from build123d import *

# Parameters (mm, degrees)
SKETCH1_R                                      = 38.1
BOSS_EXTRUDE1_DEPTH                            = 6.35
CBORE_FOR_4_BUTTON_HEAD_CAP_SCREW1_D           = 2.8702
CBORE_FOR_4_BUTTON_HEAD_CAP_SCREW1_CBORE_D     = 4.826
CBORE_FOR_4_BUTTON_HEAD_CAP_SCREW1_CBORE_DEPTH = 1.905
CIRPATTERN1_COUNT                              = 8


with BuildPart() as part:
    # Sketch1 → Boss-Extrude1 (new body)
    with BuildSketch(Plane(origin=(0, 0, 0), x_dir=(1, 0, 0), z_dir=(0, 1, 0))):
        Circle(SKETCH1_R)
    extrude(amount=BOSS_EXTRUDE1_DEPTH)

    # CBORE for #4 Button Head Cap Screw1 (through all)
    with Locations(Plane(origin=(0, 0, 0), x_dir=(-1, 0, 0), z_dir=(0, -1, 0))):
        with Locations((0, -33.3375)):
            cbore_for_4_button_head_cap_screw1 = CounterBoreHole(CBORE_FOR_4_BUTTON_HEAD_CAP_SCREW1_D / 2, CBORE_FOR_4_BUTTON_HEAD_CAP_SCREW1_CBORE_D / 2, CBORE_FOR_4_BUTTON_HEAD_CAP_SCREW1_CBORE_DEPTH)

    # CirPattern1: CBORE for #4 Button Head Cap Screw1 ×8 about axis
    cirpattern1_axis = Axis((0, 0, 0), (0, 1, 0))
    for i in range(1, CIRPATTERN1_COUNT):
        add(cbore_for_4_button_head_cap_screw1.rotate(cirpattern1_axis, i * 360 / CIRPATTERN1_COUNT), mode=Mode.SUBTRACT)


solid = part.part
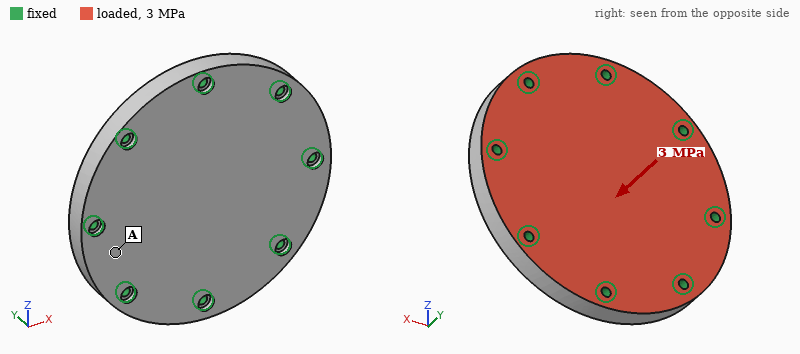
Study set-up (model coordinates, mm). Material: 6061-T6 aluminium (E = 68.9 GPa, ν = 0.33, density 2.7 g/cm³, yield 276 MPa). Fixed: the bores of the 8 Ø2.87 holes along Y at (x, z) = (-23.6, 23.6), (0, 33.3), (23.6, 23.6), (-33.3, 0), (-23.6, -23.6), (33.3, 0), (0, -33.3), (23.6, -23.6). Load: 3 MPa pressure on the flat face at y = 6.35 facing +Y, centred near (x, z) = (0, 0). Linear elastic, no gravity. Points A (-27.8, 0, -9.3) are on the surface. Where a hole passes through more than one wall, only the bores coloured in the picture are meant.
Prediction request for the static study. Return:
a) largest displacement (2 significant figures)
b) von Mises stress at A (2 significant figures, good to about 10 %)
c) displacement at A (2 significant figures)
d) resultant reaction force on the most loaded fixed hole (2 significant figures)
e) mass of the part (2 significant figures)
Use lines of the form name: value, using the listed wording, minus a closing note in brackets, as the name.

largest displacement: 70 µm
von Mises stress at A: 36 MPa
displacement at A: 16 µm
resultant reaction force on the most loaded fixed hole: 1.8 kN
mass of the part: 77 g
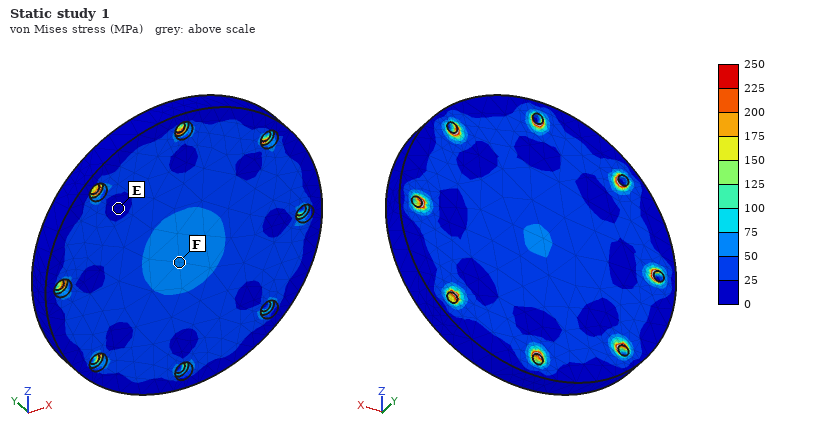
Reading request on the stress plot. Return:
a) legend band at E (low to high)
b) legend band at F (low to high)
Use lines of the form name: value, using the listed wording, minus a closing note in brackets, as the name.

legend band at E: 0 to 25 MPa
legend band at F: 50 to 75 MPa
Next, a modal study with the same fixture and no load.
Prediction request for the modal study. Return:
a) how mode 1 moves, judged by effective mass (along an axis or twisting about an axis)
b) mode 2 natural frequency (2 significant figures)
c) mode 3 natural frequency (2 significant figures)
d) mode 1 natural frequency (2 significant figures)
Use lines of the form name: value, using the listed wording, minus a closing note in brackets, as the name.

how mode 1 moves, judged by effective mass: along Y
mode 2 natural frequency: 20 kHz
mode 3 natural frequency: 20 kHz
mode 1 natural frequency: 9700 Hz
